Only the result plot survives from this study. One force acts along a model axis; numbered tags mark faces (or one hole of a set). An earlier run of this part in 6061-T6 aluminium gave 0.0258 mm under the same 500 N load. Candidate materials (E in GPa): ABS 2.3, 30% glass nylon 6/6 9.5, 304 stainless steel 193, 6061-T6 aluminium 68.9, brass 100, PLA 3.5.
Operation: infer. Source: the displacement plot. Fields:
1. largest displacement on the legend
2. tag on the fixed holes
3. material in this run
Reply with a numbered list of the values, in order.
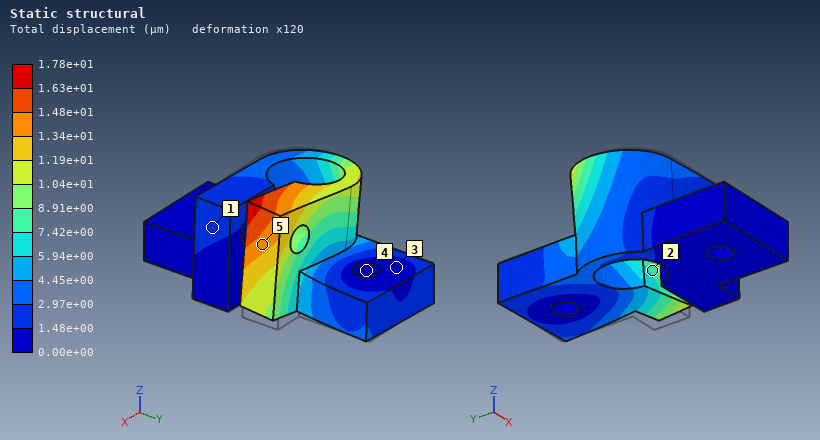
1. 1.78e+01 µm
2. 4
3. brass
